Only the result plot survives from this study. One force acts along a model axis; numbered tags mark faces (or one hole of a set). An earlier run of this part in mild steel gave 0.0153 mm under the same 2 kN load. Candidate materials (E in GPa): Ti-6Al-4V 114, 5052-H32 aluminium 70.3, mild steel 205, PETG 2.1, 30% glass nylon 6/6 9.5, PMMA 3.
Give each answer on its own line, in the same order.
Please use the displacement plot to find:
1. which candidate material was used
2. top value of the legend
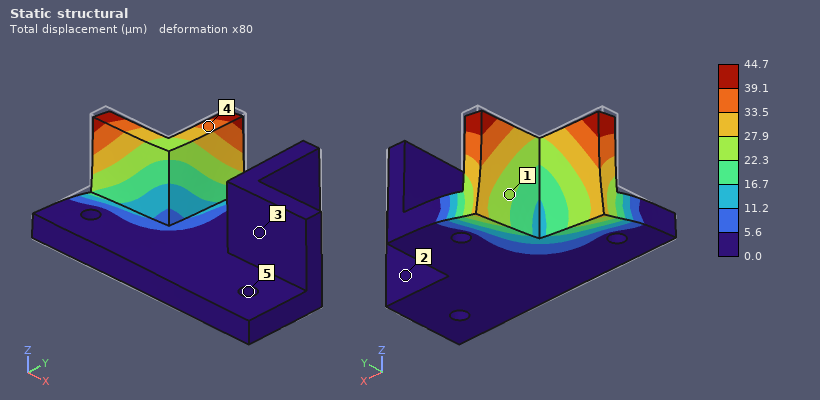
5052-H32 aluminium
44.7 µm
